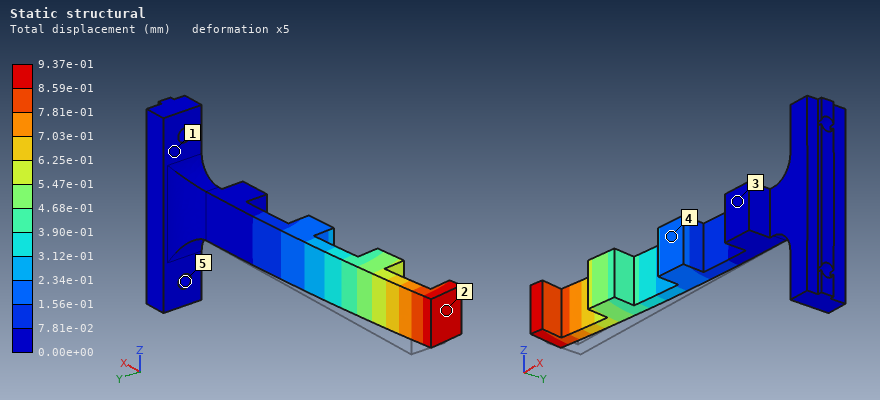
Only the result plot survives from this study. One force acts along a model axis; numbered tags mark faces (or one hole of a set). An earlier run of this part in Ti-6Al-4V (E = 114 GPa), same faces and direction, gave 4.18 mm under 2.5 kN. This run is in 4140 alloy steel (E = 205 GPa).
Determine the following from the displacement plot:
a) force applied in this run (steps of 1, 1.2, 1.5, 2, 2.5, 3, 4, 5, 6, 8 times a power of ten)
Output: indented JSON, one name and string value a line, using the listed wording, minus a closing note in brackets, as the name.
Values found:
{
  "force applied in this run": "1 kN"
}
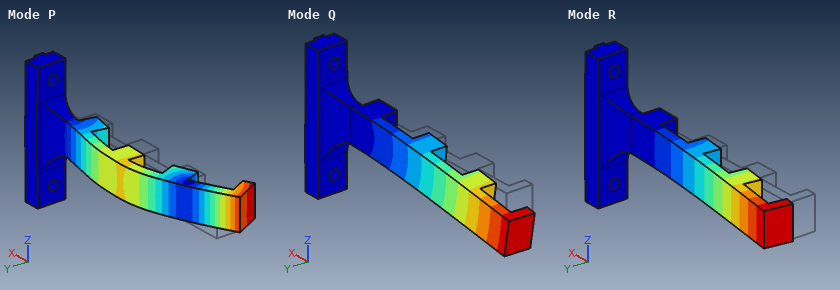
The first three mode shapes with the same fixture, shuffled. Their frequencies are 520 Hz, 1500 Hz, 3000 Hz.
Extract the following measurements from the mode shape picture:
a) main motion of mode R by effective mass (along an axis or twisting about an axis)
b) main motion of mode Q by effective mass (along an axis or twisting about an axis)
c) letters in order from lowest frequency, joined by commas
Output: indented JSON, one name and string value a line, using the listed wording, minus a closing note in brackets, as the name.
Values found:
{
  "main motion of mode R by effective mass": "along Y",
  "main motion of mode Q by effective mass": "along Z",
  "letters in order from lowest frequency, joined by commas": "R, Q, P"
}
